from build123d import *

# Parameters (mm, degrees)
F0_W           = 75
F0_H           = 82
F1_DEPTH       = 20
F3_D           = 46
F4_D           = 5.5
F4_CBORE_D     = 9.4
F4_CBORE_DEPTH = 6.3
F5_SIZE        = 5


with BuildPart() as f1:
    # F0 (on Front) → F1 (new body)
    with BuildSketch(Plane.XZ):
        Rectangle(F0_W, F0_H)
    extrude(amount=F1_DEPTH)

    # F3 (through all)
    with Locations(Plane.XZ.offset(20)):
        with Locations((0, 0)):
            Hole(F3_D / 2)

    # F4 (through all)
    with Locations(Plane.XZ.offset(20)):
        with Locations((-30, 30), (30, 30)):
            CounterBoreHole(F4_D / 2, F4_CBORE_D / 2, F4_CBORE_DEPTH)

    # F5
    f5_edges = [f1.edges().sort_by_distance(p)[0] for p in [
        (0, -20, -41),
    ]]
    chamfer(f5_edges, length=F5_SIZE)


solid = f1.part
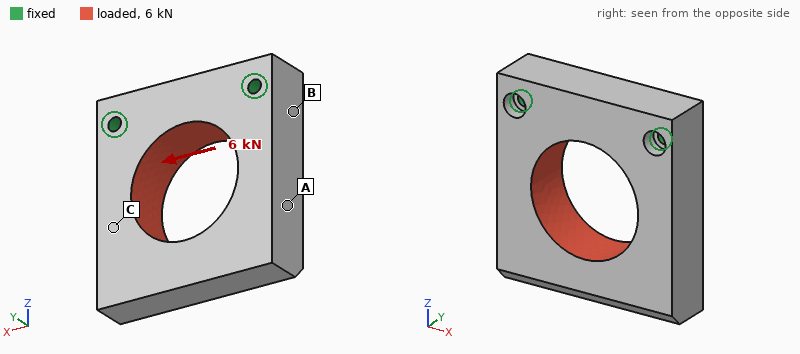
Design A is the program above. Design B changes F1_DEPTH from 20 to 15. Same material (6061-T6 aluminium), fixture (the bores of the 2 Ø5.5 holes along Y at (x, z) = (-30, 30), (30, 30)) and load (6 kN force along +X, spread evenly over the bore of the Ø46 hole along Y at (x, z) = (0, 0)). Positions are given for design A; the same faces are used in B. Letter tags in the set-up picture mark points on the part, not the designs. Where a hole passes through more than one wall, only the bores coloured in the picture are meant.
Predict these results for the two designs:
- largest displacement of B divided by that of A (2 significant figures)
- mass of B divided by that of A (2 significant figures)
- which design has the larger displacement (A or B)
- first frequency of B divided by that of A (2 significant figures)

1.2
0.75
B
0.91
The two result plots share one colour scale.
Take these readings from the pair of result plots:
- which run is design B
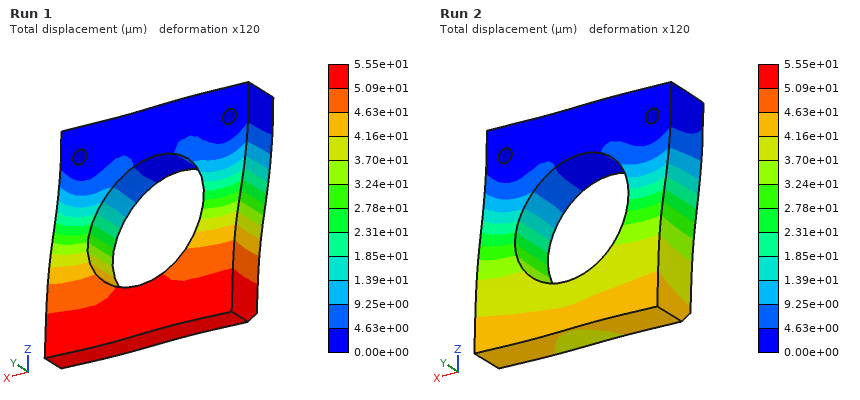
Run 1
